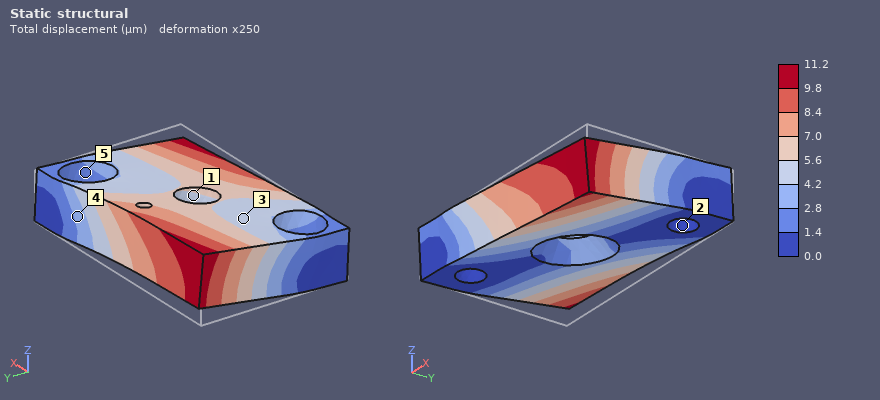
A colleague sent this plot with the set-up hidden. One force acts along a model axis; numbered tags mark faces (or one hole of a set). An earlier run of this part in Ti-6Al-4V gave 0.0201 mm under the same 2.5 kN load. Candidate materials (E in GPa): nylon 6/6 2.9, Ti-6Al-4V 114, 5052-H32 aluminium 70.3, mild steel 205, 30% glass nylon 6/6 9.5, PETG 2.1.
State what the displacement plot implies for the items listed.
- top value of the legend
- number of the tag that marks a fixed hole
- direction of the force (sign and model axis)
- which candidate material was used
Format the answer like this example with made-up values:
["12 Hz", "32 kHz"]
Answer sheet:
["11.2 µm", "2", "-Y", "mild steel"]
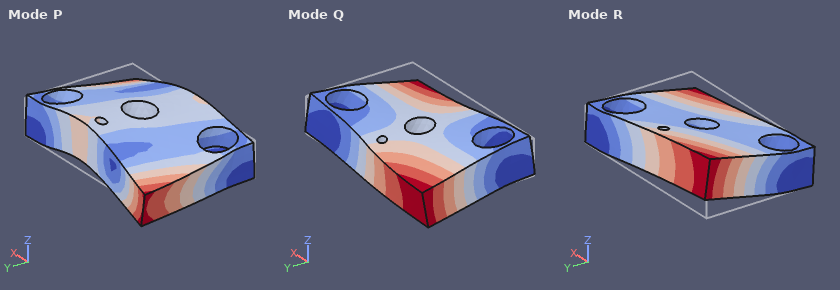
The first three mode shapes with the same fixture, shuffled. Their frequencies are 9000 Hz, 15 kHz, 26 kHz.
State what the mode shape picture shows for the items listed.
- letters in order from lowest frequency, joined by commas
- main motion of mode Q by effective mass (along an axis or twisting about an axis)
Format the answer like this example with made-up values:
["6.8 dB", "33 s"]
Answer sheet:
["R, Q, P", "along Z"]
